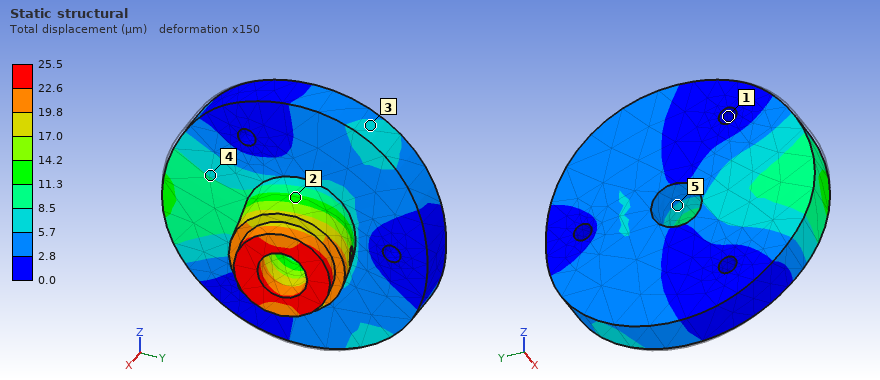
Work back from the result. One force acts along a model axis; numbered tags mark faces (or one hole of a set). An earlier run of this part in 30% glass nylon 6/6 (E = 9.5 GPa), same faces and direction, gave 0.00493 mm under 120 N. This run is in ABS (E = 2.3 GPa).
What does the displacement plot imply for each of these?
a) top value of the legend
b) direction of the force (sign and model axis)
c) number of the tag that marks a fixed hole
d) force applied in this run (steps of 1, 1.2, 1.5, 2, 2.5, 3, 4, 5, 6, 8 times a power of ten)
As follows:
25.5 µm
+Y
1
150 N
